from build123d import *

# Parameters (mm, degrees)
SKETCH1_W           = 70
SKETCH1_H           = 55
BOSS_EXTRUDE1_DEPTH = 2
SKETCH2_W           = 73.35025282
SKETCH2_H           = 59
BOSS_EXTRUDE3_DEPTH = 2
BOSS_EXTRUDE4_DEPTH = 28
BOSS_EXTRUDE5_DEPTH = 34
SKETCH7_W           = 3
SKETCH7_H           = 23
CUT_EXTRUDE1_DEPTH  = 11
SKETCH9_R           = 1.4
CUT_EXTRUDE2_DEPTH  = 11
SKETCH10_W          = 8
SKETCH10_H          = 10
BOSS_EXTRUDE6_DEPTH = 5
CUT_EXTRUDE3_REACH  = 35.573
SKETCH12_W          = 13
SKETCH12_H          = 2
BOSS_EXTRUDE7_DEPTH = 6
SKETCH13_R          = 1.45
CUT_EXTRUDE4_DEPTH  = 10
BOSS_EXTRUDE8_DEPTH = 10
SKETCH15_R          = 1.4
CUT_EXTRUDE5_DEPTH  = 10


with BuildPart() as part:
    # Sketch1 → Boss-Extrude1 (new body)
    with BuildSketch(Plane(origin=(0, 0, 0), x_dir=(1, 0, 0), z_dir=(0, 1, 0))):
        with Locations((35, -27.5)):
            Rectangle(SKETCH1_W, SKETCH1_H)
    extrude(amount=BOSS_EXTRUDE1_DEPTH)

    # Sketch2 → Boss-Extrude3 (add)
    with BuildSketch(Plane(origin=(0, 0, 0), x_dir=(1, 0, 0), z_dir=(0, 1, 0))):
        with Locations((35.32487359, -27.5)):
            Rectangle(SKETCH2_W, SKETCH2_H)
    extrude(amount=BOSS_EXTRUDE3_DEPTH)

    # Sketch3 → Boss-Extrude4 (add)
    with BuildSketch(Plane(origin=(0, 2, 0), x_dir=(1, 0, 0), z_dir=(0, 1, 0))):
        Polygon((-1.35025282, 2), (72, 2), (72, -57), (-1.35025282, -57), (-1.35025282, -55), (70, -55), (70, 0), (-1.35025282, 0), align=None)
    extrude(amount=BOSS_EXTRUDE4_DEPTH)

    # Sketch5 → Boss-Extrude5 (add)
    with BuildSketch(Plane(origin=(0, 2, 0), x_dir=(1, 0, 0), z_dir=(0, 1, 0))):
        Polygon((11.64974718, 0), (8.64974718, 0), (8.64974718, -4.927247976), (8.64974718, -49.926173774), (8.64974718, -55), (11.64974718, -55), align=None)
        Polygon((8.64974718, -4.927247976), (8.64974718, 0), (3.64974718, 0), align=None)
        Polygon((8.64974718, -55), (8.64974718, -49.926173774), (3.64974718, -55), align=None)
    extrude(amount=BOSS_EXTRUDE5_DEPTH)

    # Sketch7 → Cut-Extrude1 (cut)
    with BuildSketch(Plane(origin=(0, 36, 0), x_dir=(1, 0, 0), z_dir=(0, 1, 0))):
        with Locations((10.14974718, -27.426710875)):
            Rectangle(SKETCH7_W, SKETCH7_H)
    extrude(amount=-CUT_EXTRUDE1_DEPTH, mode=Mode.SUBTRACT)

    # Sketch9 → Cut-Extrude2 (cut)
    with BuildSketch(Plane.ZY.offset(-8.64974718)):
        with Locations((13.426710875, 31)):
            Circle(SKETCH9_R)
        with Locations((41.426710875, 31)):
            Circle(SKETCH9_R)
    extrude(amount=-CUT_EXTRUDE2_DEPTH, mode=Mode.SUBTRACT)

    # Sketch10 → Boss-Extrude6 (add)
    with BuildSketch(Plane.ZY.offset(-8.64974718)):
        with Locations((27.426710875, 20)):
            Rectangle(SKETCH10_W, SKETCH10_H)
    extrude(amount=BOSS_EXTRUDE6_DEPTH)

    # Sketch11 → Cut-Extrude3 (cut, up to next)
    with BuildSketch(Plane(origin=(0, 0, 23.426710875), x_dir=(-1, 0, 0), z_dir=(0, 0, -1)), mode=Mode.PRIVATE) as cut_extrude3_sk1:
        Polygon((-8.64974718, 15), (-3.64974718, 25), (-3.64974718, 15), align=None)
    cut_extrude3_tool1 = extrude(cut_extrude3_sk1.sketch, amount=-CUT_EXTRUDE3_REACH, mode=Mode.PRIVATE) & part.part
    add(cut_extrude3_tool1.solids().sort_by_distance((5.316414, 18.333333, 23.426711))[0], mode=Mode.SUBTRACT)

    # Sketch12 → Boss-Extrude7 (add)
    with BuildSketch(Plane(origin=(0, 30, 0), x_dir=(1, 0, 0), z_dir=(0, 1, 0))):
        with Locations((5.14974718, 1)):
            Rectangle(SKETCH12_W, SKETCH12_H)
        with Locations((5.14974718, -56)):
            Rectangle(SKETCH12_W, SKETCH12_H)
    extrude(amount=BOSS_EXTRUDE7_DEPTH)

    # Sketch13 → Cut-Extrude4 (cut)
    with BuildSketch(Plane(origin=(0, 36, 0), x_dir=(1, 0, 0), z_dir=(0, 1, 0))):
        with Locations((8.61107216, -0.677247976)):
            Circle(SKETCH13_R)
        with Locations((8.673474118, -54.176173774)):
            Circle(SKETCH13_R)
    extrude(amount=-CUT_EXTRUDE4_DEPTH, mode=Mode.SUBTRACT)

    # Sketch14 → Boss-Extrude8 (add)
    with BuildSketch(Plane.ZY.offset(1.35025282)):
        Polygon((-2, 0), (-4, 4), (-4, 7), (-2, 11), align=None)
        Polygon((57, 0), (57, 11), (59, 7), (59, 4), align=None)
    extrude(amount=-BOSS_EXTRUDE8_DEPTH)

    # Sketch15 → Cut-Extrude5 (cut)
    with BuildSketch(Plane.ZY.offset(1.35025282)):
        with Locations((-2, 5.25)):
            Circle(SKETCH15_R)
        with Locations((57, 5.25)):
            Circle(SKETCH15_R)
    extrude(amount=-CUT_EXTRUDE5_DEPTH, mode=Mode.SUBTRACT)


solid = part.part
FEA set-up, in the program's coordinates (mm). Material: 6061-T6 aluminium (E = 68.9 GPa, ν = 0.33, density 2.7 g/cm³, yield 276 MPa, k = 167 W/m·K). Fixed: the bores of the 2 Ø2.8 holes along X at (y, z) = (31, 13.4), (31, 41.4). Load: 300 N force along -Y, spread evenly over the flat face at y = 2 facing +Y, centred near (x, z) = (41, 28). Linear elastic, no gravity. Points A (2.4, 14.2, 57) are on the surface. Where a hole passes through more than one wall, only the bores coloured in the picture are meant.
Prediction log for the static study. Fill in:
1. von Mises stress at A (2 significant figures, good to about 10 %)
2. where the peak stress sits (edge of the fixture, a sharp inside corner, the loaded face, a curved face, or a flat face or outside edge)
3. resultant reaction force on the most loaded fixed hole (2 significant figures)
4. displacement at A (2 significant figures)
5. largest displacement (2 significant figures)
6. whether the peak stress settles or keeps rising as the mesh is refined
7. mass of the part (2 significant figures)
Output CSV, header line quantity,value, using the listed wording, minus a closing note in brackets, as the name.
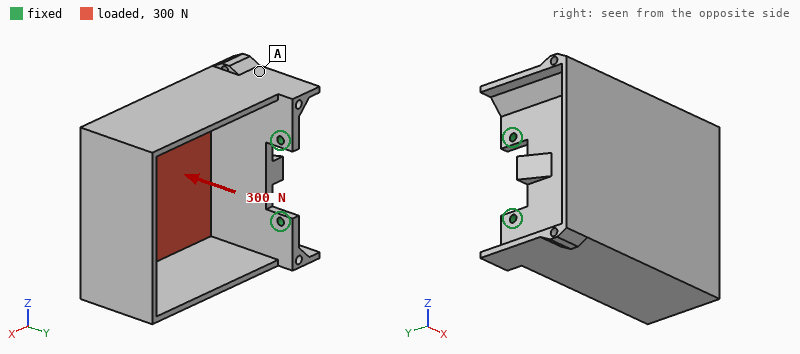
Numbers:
quantity,value
von Mises stress at A,20 MPa
where the peak stress sits,edge of the fixture
resultant reaction force on the most loaded fixed hole,150 N
displacement at A,0.20 mm
largest displacement,0.89 mm
whether the peak stress settles or keeps rising as the mesh is refined,keeps rising
mass of the part,71 g
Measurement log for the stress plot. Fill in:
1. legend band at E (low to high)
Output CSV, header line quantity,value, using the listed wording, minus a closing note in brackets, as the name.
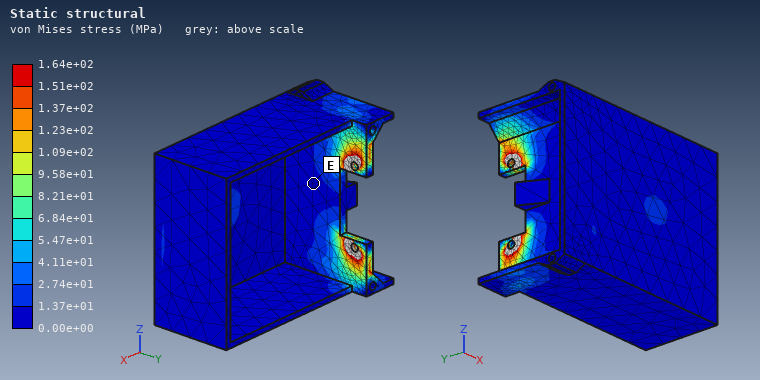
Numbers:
quantity,value
legend band at E,0.00e+00 to 1.37e+01 MPa
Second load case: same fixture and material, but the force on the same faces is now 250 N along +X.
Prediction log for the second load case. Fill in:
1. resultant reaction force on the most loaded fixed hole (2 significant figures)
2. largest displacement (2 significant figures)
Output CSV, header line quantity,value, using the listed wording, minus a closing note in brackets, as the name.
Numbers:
quantity,value
resultant reaction force on the most loaded fixed hole,130 N
largest displacement,0.63 mm
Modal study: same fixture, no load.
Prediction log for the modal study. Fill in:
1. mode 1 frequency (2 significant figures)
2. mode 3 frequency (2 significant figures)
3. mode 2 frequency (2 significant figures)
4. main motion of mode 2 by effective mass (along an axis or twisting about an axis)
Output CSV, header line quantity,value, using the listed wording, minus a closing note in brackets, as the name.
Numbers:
quantity,value
mode 1 frequency,410 Hz
mode 3 frequency,2100 Hz
mode 2 frequency,480 Hz
main motion of mode 2 by effective mass,along Z
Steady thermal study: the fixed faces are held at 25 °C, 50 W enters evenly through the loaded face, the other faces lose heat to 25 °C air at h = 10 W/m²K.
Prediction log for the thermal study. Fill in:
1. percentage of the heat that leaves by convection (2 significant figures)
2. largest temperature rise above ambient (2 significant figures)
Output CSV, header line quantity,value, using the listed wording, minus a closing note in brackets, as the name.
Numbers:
quantity,value
percentage of the heat that leaves by convection,22 %
largest temperature rise above ambient,74 K
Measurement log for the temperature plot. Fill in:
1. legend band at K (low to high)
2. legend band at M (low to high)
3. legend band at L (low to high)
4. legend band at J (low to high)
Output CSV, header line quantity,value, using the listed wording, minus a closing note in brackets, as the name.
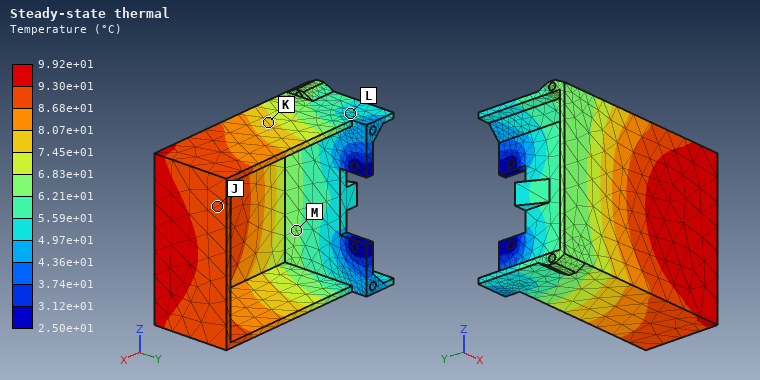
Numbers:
quantity,value
legend band at K,7.45e+01 to 8.07e+01 °C
legend band at M,6.21e+01 to 6.83e+01 °C
legend band at L,4.97e+01 to 5.59e+01 °C
legend band at J,8.68e+01 to 9.30e+01 °C
